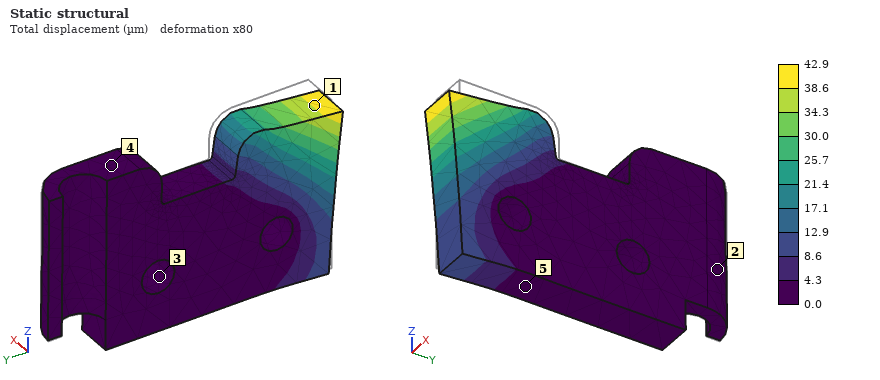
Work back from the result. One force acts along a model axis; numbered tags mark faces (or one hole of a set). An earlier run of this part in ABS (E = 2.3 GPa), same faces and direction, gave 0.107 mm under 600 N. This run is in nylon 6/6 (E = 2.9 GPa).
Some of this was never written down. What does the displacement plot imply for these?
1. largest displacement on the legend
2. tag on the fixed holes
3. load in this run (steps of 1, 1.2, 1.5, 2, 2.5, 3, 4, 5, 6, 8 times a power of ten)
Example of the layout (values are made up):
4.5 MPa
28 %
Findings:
42.9 µm
3
300 N
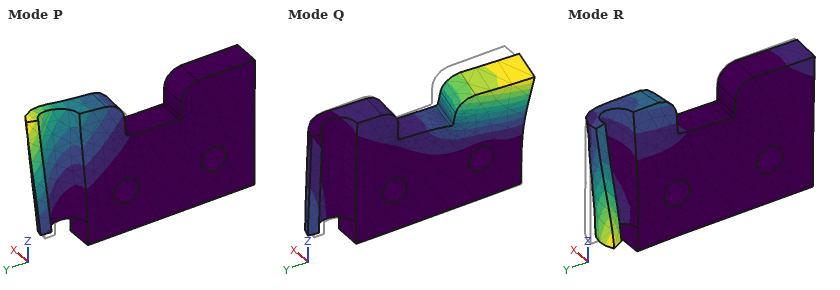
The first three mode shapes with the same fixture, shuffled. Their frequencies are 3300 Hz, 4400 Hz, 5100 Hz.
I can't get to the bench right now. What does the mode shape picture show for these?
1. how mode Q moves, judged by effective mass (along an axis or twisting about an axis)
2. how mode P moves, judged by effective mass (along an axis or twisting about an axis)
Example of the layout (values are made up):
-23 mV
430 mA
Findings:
along X
along X
